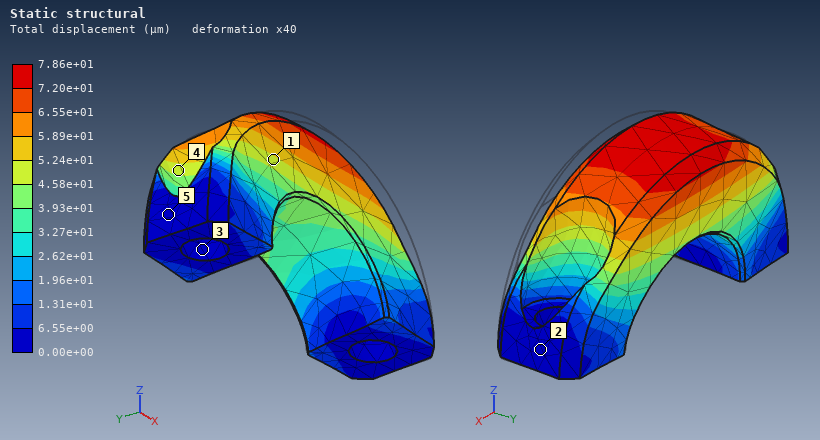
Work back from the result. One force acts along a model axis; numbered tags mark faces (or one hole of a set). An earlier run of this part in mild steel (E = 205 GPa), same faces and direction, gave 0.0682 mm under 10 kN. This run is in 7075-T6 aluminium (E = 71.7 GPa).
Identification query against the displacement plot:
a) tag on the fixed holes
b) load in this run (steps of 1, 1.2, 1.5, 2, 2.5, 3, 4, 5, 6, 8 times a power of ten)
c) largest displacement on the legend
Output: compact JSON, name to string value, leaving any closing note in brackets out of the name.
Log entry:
{"tag on the fixed holes": "3", "load in this run": "4 kN", "largest displacement on the legend": "7.86e+01 µm"}
